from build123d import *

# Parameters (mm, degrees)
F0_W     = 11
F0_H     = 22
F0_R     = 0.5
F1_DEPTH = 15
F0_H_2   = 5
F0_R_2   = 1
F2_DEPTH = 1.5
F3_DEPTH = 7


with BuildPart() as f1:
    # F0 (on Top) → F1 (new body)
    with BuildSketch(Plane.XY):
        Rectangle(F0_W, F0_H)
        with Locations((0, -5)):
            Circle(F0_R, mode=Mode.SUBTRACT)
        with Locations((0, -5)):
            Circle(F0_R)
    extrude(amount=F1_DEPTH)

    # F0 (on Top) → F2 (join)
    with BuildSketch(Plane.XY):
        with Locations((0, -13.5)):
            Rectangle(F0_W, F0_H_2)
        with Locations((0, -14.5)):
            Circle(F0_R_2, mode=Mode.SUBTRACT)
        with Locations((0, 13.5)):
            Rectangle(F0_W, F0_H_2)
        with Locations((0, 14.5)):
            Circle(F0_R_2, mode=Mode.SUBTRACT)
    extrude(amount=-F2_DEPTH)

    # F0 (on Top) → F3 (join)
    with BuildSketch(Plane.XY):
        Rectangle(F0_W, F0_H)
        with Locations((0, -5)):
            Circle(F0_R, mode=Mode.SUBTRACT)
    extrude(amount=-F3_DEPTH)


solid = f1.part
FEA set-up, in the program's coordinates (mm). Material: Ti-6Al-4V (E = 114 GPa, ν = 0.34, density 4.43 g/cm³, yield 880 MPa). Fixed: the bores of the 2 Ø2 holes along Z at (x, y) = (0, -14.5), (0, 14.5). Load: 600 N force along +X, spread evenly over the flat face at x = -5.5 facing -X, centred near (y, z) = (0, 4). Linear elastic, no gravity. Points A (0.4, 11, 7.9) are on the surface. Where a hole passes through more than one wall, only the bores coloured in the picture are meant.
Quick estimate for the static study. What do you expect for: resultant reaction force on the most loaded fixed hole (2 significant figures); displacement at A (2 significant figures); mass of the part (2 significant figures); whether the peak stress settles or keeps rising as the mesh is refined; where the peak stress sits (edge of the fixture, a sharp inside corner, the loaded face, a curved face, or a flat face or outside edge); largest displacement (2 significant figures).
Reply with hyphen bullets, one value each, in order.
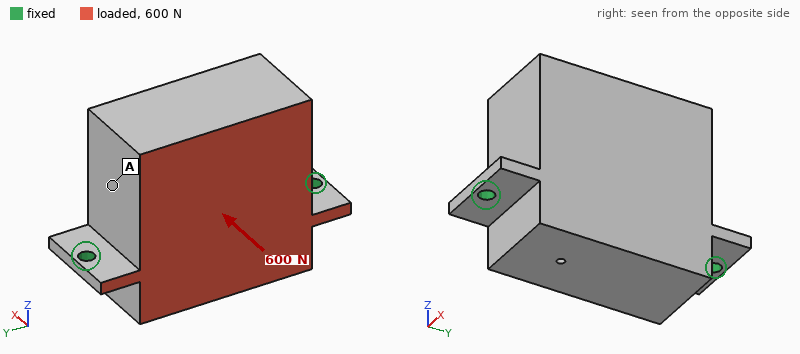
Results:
- 300 N
- 0.068 mm
- 24 g
- keeps rising
- edge of the fixture
- 0.13 mm
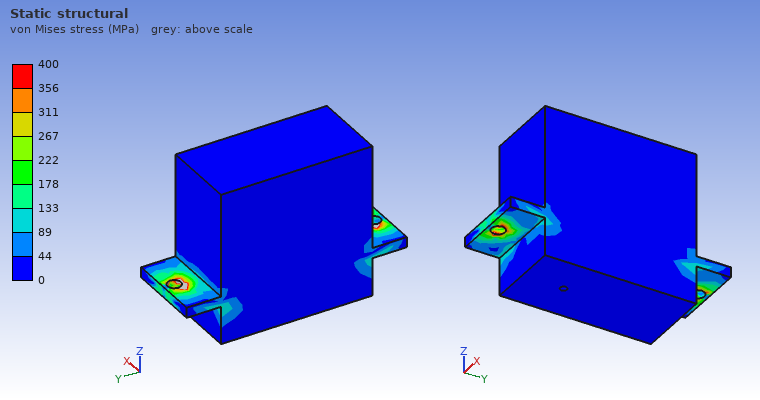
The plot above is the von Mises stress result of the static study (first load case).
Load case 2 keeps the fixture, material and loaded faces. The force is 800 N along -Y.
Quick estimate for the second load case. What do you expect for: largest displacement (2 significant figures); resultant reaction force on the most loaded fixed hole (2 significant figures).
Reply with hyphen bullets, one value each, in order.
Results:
- 8.6 µm
- 450 N
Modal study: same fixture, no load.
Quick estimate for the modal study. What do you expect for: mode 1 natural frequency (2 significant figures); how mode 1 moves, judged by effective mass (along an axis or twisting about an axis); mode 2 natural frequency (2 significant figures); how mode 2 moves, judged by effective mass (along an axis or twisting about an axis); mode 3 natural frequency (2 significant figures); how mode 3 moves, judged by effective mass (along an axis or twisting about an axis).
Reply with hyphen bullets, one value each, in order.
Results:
- 2300 Hz
- along X
- 9200 Hz
- along Z
- 11 kHz
- along Y
